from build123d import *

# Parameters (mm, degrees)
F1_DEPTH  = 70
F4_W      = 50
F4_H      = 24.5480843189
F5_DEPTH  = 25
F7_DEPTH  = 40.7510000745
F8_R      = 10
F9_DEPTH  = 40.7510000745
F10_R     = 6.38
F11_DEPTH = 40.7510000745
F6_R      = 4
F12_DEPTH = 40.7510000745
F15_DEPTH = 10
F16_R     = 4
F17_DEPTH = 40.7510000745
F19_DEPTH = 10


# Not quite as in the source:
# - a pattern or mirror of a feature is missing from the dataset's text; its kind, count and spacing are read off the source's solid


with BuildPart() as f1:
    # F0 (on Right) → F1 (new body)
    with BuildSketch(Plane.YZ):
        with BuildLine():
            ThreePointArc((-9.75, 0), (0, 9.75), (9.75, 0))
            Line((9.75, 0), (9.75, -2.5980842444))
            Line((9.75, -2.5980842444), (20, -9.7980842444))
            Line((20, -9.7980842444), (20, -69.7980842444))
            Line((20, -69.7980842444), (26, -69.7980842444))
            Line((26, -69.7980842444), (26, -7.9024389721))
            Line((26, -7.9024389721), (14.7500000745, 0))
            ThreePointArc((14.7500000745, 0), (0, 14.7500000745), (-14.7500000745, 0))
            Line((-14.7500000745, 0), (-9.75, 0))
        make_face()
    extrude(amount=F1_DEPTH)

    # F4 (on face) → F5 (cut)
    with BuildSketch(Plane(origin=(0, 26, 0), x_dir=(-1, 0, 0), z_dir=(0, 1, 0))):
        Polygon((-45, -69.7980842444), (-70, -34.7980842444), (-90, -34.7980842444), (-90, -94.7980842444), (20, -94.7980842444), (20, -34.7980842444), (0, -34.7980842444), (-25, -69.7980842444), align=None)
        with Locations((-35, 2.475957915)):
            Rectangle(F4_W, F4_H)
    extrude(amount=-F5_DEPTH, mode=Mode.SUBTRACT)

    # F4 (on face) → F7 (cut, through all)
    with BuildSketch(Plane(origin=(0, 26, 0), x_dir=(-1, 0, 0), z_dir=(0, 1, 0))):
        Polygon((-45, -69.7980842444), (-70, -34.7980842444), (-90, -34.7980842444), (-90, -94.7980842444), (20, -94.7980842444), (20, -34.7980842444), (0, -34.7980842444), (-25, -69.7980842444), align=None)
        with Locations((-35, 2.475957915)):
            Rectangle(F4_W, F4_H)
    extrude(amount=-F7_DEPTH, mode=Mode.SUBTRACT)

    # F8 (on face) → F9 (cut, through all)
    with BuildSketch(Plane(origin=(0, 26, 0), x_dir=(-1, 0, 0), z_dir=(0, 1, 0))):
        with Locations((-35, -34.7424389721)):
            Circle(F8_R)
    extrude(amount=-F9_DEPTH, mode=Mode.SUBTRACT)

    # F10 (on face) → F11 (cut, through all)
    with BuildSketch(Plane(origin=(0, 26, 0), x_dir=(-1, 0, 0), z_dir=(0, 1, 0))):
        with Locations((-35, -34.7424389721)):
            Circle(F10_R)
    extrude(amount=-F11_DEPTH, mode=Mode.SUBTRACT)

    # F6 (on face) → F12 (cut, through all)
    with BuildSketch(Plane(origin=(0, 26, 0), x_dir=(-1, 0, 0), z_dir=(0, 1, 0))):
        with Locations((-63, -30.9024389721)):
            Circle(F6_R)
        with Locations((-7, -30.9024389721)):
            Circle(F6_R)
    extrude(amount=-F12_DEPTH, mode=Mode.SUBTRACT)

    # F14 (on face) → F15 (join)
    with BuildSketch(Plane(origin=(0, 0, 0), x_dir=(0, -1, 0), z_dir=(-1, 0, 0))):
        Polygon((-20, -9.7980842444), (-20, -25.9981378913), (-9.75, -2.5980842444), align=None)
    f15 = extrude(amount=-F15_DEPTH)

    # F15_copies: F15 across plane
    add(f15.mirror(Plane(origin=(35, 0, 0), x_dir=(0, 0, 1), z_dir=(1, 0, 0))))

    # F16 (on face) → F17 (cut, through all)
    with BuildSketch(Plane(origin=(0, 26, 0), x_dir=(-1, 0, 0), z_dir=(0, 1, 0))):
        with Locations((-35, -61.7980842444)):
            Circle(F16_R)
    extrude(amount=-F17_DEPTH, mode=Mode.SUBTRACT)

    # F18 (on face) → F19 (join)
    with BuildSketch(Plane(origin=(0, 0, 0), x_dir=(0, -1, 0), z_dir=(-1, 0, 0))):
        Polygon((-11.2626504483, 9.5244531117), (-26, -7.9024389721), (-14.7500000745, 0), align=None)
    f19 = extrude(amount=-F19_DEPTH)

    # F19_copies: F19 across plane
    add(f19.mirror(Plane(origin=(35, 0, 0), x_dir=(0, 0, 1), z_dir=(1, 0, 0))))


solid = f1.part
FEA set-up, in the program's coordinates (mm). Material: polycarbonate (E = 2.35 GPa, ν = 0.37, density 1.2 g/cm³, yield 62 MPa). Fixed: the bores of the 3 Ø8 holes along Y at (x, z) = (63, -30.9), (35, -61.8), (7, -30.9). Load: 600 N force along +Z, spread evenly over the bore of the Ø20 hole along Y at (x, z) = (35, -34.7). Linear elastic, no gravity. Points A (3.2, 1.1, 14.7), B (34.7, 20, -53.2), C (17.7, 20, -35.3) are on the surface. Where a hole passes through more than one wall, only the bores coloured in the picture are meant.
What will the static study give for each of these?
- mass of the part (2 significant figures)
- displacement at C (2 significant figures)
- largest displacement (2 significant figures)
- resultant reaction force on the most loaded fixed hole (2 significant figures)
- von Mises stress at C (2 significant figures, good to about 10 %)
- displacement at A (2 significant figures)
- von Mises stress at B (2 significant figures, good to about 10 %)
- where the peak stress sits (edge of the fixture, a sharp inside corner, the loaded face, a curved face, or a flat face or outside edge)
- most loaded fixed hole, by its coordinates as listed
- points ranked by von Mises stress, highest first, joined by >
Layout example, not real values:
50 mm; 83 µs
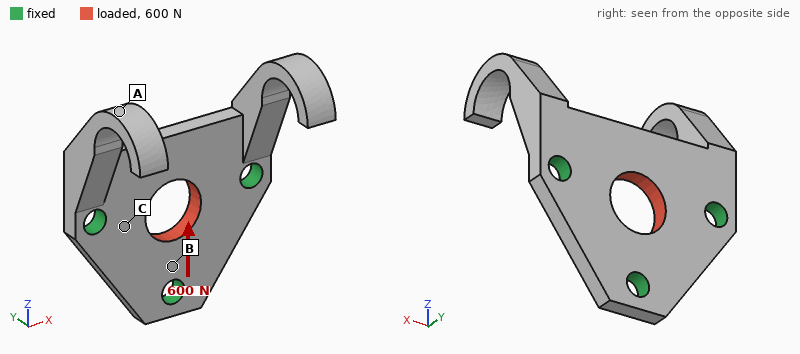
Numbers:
30 g; 15 µm; 40 µm; 250 N; 1.2 MPa; 36 µm; 3.0 MPa; edge of the fixture; (35, -61.8); B > C > A
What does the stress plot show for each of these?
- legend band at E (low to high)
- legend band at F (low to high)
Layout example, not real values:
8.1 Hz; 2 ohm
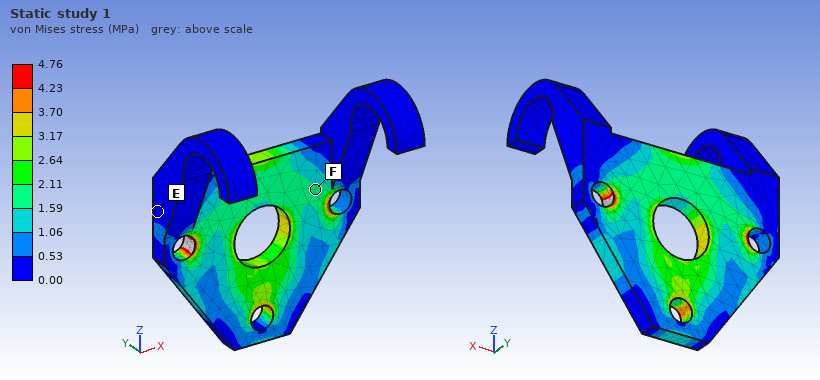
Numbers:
0.00 to 0.53 MPa; 1.59 to 2.11 MPa
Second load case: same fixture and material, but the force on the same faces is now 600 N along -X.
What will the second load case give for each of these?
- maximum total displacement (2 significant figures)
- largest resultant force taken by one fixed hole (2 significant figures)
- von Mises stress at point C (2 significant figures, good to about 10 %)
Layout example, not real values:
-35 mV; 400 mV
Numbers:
24 µm; 240 N; 2.3 MPa
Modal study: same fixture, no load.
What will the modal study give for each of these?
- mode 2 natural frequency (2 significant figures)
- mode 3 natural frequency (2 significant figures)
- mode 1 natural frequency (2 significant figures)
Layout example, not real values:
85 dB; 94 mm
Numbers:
620 Hz; 770 Hz; 610 Hz
